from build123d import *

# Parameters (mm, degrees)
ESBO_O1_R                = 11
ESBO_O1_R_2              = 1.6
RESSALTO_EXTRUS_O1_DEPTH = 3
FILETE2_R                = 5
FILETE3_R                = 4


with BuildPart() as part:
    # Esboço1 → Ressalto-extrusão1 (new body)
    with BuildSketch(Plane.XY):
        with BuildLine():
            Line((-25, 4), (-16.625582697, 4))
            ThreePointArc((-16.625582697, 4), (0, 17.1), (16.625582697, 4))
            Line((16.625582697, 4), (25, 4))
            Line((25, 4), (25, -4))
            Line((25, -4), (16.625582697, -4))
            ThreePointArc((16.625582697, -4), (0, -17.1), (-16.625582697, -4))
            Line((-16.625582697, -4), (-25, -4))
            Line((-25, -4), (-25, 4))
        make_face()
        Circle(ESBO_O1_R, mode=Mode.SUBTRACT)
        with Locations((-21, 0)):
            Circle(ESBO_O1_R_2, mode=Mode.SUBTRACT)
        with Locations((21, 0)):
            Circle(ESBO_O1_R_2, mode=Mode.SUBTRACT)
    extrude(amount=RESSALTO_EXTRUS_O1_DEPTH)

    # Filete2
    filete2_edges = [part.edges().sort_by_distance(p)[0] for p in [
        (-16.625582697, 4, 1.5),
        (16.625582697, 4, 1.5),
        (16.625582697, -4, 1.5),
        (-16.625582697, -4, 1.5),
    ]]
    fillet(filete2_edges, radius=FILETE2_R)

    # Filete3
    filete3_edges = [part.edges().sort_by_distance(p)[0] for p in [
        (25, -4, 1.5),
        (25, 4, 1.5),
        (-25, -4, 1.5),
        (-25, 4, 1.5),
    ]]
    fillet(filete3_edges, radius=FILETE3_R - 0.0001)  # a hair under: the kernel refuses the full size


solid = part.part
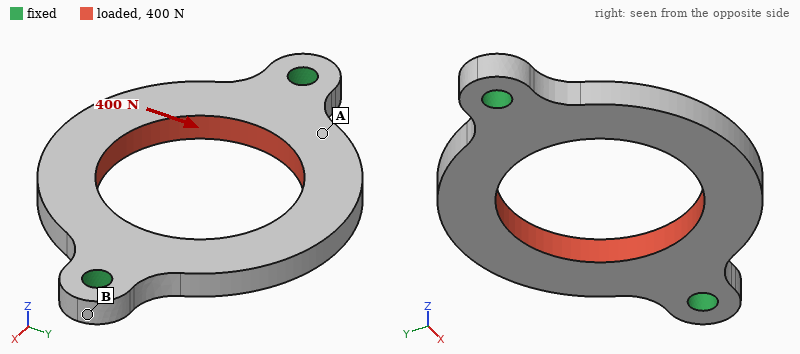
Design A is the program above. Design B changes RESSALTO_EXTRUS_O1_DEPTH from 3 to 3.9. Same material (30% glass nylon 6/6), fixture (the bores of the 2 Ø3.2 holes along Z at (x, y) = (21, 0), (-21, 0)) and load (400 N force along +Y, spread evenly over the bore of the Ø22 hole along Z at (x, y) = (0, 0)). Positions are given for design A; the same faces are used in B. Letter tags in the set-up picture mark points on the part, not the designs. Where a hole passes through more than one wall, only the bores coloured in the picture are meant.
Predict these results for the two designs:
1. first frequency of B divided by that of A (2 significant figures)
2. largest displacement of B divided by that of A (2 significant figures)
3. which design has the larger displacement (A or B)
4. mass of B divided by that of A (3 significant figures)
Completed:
1.2
0.77
A
1.30
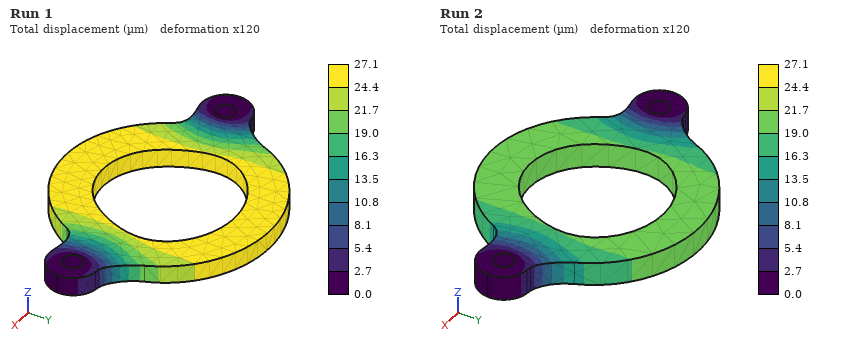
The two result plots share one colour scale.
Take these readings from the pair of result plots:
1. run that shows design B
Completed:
Run 2
